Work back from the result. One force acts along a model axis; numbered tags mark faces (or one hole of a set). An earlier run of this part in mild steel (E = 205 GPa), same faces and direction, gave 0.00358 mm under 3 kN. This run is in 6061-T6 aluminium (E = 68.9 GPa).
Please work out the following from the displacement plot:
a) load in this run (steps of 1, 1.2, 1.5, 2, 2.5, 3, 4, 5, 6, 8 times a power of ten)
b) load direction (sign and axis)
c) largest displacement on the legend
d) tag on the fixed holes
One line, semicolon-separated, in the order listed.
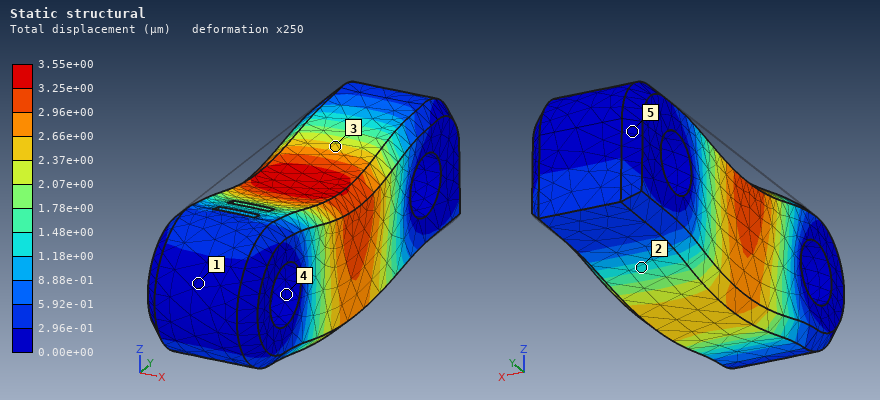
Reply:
1 kN; -Z; 3.55e+00 µm; 4
